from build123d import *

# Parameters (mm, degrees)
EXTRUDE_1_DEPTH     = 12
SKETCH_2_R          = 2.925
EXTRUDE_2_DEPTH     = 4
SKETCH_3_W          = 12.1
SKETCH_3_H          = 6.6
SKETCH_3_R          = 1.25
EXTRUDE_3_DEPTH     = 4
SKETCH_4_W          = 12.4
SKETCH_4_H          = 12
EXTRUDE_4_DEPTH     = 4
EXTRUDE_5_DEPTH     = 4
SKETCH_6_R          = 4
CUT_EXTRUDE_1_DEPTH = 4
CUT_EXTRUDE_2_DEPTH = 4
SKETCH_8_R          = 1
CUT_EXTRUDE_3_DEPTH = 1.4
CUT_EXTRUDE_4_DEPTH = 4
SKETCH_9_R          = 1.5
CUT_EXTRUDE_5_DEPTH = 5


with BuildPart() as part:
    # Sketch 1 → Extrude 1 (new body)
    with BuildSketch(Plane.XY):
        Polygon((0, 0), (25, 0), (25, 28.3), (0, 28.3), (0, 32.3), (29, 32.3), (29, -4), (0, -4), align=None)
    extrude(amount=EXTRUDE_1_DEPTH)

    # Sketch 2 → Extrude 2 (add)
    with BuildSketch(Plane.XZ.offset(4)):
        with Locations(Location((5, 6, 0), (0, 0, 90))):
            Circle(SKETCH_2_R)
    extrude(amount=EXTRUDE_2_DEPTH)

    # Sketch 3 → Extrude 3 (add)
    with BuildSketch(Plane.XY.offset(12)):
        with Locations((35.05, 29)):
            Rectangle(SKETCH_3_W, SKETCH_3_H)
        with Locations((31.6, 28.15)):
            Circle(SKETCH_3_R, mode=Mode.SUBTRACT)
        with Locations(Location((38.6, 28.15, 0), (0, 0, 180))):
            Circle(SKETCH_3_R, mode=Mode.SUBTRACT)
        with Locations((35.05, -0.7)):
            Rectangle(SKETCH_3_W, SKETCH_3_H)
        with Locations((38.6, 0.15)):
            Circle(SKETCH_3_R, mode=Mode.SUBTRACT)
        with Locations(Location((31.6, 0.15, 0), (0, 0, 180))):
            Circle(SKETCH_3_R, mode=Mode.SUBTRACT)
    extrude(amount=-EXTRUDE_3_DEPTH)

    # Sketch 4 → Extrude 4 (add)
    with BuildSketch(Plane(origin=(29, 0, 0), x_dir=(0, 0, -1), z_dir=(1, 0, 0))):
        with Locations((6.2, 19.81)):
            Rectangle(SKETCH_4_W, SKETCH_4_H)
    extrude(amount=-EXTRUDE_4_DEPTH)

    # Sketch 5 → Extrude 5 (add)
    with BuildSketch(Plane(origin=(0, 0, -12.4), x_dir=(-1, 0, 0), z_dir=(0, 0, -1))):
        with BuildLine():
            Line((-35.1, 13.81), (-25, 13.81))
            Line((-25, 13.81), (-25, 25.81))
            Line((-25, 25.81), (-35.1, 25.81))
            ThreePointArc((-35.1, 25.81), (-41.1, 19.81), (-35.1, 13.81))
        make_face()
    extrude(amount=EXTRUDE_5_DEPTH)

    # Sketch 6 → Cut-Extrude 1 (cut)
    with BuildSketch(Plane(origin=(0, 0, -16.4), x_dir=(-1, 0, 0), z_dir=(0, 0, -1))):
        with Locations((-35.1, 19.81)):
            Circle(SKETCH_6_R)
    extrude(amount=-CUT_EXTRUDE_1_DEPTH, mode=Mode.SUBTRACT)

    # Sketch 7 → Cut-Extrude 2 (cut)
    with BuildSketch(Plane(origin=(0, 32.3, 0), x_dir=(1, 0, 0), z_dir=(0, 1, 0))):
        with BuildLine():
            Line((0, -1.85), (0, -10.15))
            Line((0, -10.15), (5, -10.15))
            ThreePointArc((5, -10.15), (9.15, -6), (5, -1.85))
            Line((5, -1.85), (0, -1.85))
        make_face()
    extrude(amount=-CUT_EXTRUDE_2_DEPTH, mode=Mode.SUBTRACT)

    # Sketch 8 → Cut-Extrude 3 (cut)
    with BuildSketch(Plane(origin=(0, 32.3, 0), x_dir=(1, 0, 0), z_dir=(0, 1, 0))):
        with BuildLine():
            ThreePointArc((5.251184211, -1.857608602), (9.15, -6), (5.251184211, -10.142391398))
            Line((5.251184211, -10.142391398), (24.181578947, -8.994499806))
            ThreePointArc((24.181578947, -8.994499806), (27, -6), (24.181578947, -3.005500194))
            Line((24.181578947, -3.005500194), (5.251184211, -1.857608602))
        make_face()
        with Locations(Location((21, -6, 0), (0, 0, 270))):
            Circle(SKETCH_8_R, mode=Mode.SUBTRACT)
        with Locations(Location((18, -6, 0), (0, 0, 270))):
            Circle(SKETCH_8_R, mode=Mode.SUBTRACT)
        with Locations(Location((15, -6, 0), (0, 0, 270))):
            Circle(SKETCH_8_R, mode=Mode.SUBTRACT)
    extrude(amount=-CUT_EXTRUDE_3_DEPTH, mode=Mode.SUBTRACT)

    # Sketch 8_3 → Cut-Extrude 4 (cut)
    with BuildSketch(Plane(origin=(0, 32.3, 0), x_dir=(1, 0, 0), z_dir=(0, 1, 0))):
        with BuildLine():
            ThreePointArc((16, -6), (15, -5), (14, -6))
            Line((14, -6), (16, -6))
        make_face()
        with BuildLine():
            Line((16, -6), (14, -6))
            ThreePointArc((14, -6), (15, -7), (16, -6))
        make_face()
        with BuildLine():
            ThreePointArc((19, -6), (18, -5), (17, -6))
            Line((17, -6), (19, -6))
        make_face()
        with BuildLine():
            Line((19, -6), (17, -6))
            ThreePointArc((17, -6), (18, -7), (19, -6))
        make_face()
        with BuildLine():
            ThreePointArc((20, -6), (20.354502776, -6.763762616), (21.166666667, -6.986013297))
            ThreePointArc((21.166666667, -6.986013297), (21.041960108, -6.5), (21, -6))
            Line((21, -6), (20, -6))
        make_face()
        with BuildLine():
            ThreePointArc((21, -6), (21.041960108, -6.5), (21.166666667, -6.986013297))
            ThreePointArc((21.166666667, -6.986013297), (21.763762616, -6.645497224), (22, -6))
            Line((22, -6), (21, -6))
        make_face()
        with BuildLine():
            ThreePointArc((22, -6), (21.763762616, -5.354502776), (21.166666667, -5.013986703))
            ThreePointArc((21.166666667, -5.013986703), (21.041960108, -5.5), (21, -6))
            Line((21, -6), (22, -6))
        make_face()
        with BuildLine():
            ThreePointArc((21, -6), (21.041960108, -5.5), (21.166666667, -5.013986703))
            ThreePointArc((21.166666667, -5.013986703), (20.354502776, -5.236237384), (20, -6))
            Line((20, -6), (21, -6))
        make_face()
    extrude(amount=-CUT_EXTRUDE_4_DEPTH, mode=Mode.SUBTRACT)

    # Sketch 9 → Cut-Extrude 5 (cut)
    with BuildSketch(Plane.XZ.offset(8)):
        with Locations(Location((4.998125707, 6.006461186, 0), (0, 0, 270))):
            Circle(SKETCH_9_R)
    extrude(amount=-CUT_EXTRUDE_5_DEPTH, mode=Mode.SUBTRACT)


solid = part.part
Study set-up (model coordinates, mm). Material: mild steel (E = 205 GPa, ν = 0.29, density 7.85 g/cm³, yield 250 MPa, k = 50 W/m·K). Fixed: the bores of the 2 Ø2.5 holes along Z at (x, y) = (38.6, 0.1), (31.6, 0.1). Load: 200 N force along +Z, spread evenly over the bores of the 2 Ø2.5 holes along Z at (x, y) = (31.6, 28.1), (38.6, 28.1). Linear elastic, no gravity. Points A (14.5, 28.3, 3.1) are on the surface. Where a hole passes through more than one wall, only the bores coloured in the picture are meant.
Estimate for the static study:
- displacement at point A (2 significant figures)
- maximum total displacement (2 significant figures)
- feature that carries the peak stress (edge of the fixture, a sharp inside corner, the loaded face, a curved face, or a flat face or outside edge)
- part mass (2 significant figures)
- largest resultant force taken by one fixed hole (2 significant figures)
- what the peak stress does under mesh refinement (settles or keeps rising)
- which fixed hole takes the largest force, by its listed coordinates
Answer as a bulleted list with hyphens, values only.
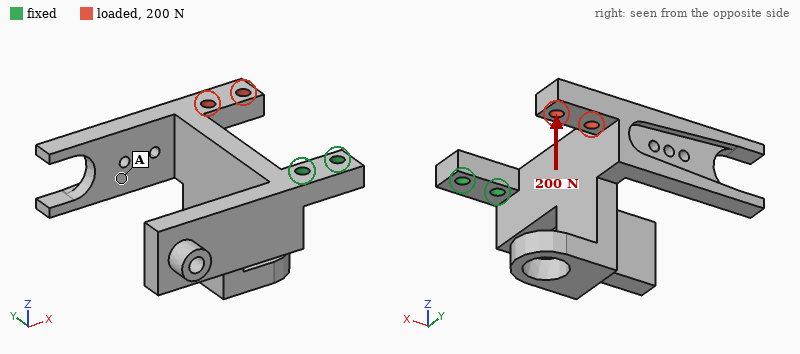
- 0.052 mm
- 0.16 mm
- edge of the fixture
- 42 g
- 170 N
- keeps rising
- (31.6, 0.1)
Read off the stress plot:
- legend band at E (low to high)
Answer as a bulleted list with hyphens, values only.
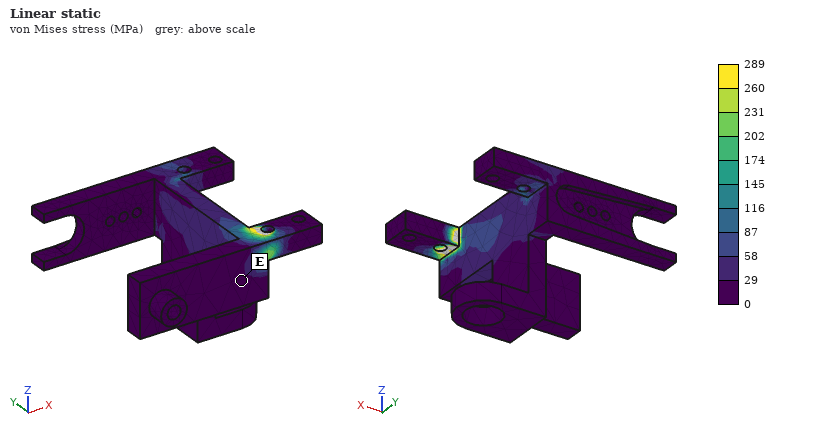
- 0 to 29 MPa
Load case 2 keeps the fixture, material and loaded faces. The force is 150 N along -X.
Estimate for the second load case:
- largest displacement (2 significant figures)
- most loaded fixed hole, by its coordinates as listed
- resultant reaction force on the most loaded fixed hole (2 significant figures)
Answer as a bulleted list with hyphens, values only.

- 0.21 mm
- (31.6, 0.1)
- 440 N
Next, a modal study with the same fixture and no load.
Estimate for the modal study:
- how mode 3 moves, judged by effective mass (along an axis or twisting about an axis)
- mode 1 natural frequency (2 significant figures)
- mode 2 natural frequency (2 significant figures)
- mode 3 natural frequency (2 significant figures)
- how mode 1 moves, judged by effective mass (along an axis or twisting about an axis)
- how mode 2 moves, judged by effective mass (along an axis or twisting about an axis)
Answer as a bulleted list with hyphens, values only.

- twisting about Y
- 1100 Hz
- 1500 Hz
- 1900 Hz
- along X
- along Z
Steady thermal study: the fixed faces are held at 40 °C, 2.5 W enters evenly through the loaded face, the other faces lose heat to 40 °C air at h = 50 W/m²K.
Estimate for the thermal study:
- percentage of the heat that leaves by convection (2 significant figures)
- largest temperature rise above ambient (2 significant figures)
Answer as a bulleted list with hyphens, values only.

- 68 %
- 31 K
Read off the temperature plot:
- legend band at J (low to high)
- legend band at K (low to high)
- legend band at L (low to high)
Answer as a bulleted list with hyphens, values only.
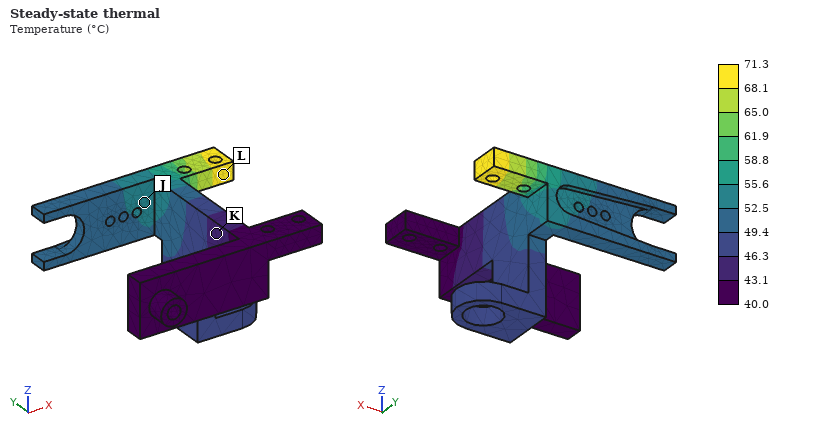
- 52.5 to 55.6 °C
- 43.1 to 46.3 °C
- 68.1 to 71.3 °C
